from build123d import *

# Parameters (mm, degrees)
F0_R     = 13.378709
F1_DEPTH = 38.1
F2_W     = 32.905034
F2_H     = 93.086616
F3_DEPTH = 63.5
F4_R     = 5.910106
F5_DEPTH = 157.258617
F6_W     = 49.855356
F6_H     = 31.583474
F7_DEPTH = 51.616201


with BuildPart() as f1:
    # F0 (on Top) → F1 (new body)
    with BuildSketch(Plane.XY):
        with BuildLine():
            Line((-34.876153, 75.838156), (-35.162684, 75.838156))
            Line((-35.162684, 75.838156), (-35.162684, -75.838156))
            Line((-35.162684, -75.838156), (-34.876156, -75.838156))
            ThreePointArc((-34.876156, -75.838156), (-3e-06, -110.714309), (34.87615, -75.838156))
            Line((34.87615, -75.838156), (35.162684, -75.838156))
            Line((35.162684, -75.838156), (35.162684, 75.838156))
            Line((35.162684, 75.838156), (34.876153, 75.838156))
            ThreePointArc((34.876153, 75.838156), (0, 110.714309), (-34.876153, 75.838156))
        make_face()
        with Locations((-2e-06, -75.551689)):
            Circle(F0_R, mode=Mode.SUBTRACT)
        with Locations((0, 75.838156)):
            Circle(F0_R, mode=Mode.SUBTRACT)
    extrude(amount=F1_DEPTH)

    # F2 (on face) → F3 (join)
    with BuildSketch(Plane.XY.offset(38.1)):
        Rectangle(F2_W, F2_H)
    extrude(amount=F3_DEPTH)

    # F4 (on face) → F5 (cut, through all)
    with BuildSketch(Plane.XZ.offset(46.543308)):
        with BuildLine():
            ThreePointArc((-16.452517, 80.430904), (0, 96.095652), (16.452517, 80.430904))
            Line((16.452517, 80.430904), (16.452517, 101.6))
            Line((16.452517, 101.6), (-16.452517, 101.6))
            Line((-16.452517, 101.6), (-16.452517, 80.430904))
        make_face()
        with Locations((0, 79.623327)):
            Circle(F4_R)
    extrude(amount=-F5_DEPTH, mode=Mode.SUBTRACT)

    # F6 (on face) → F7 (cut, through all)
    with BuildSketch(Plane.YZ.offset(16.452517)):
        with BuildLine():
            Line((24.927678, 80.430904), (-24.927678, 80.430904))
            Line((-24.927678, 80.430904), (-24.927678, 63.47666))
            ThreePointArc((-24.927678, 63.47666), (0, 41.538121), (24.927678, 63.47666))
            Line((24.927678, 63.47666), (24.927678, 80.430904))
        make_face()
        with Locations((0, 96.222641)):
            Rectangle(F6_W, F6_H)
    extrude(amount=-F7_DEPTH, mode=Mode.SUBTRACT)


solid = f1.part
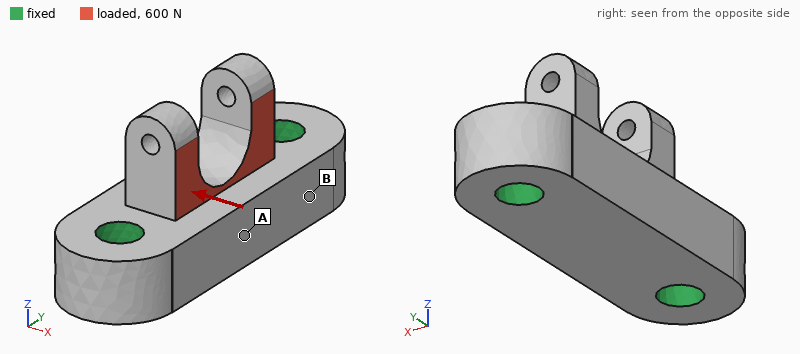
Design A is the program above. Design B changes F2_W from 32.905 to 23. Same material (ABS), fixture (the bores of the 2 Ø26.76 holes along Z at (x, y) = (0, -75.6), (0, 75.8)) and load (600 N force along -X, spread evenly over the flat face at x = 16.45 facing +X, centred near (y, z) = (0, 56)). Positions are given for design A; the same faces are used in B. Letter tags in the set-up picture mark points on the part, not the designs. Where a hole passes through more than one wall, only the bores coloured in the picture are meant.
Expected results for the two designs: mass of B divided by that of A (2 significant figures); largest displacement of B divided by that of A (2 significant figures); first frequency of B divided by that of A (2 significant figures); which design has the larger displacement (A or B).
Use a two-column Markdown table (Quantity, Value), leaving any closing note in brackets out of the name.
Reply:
| Quantity | Value |
|---|---|
| mass of B divided by that of A | 0.96 |
| largest displacement of B divided by that of A | 2.3 |
| first frequency of B divided by that of A | 0.92 |
| which design has the larger displacement | B |
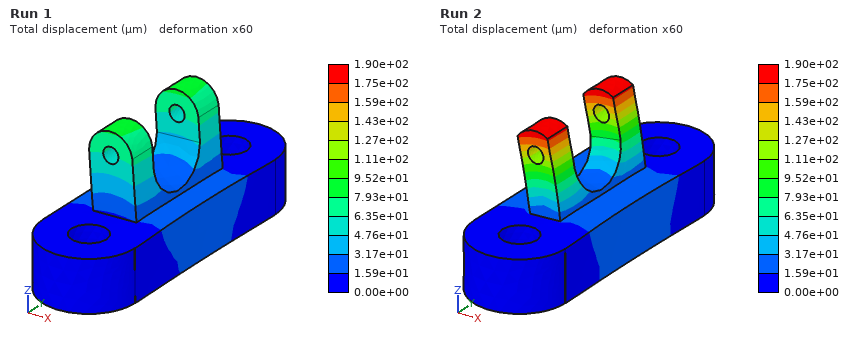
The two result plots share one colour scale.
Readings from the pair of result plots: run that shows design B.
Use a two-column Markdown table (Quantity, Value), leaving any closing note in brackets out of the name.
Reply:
| Quantity | Value |
|---|---|
| run that shows design B | Run 2 |
